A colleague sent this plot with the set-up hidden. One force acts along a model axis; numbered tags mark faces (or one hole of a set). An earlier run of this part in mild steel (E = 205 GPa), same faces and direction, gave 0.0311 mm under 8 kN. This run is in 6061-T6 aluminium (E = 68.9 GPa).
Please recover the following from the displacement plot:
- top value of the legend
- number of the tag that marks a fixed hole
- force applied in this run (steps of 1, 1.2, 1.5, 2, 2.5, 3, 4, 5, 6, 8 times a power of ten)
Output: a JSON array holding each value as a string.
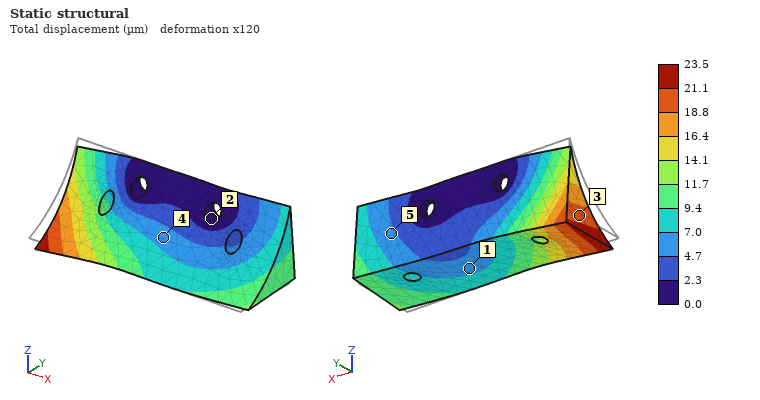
["23.5 µm", "2", "2 kN"]
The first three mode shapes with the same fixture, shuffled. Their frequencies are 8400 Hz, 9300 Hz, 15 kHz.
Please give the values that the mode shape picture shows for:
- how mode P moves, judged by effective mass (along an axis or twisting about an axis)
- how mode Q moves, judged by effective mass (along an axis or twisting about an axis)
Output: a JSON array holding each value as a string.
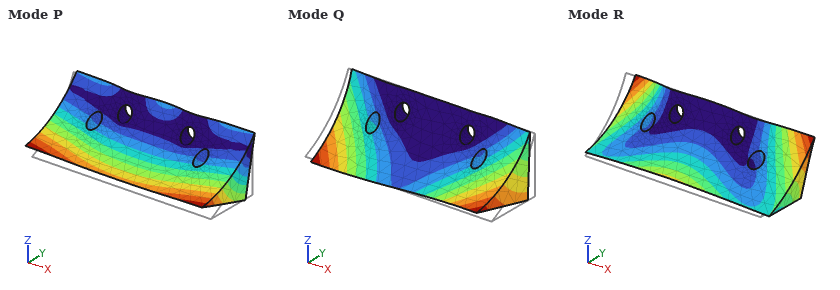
["along Y", "twisting about Z"]
